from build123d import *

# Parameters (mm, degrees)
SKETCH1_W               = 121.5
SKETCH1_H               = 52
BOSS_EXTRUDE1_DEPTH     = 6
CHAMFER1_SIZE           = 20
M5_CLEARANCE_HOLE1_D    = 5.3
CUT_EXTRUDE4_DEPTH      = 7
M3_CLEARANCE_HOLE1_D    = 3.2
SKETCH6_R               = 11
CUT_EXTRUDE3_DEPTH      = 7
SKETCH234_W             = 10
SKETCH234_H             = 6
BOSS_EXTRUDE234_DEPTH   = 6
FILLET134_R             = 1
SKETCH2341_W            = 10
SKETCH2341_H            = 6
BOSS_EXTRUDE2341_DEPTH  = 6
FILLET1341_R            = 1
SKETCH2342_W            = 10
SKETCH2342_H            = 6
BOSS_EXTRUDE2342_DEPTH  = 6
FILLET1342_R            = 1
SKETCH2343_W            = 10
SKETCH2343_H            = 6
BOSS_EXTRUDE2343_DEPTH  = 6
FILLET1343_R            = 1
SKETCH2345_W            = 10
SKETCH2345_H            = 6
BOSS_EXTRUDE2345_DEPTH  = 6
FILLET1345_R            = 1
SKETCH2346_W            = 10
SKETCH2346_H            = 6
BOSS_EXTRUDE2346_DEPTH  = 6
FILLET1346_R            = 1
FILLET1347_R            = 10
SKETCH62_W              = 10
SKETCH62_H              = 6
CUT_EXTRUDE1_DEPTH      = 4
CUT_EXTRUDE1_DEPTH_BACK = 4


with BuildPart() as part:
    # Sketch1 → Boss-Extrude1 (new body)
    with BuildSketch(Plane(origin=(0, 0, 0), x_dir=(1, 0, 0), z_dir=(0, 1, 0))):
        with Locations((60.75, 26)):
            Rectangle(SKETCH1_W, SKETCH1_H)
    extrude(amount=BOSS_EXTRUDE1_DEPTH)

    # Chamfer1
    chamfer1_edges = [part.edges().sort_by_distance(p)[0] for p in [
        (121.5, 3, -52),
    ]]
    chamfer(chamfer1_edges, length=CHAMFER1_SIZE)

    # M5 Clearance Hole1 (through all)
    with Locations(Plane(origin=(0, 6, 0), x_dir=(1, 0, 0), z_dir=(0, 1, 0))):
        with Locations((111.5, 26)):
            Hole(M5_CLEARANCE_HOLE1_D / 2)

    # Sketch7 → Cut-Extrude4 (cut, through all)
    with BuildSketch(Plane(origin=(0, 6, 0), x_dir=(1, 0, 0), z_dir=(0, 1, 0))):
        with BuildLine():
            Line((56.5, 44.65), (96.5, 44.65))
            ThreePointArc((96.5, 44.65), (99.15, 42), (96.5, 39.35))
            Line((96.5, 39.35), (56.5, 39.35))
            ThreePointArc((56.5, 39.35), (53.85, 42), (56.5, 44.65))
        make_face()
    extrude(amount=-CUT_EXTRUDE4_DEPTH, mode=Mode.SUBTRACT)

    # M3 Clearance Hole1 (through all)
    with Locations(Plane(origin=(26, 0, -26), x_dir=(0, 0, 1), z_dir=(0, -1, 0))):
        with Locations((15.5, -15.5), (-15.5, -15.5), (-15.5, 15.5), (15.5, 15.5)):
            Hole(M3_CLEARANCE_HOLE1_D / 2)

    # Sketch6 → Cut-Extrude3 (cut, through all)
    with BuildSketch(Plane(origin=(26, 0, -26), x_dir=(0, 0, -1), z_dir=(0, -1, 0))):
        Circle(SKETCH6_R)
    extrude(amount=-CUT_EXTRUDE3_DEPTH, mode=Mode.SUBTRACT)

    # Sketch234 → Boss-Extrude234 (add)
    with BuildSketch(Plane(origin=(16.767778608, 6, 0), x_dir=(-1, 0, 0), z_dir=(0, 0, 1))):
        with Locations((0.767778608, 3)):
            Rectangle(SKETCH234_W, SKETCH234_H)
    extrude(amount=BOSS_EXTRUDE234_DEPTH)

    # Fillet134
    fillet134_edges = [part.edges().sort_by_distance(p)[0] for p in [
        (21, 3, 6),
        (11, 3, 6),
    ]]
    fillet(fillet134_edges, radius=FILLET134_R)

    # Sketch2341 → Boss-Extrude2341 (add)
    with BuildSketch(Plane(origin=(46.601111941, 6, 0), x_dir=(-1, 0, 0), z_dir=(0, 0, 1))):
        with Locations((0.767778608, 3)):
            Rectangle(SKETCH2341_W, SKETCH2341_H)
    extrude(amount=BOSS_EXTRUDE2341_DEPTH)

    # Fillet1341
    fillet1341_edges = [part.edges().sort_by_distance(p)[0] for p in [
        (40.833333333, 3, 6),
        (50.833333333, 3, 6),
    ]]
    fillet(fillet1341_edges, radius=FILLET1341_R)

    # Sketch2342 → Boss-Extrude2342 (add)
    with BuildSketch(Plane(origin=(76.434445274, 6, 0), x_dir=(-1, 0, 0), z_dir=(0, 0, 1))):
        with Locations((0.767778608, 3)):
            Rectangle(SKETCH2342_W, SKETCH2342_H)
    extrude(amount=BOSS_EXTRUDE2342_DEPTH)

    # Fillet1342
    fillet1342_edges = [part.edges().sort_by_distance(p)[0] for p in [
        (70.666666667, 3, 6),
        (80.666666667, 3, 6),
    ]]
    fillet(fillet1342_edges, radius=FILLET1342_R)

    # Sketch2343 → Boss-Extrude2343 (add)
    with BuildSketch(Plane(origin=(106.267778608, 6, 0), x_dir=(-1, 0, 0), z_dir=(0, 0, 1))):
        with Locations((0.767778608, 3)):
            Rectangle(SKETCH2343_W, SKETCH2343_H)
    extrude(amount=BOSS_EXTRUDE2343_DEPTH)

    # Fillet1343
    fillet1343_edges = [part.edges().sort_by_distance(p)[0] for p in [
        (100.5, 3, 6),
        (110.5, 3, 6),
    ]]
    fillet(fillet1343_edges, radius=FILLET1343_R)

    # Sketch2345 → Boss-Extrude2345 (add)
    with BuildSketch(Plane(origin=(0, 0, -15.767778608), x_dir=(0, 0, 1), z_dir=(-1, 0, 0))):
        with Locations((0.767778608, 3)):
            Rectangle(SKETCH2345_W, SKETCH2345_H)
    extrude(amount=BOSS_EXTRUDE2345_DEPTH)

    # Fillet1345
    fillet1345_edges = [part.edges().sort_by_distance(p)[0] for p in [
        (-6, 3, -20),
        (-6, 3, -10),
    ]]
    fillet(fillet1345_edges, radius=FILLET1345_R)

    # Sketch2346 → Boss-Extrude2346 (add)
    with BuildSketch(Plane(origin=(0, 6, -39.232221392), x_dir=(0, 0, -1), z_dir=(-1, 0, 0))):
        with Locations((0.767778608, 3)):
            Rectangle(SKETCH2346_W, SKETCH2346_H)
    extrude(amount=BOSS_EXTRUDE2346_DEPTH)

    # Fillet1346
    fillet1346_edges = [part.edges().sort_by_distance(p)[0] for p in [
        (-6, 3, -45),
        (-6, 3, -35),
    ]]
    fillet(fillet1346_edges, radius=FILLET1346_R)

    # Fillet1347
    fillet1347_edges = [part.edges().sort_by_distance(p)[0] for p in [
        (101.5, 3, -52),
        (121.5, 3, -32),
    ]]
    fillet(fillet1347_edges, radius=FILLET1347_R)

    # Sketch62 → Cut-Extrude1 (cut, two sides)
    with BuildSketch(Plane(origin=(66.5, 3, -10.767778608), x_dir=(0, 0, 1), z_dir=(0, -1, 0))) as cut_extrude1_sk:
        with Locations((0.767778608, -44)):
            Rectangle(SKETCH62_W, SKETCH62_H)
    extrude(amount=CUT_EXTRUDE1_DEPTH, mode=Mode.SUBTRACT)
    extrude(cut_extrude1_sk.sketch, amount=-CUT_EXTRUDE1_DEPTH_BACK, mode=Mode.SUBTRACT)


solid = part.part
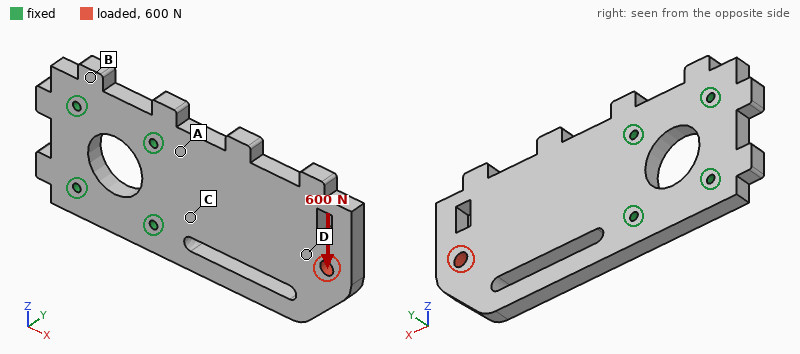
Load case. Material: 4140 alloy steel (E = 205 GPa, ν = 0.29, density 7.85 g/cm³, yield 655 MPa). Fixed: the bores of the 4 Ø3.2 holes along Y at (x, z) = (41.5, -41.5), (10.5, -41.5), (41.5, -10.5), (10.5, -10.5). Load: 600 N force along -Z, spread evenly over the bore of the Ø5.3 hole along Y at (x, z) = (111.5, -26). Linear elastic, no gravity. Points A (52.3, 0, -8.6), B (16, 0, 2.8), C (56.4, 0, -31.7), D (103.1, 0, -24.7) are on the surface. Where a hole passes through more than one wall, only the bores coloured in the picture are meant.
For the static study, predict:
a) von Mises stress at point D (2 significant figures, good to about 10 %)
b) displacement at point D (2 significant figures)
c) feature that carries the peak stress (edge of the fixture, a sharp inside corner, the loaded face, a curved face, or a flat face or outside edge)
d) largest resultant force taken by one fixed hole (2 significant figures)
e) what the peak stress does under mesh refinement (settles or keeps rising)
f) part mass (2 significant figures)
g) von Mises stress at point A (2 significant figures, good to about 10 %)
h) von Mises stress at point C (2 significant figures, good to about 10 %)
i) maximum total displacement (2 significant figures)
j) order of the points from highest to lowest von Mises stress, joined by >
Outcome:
4.4 MPa
8.6 µm
edge of the fixture
1.1 kN
keeps rising
270 g
11 MPa
8.0 MPa
12 µm
A > C > D > B
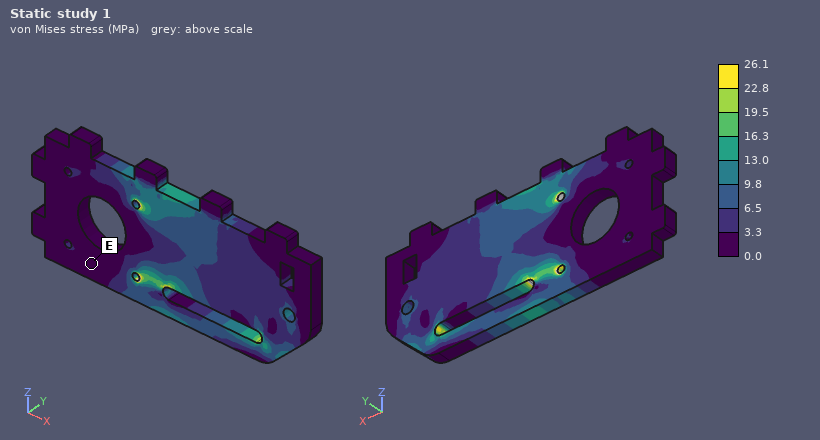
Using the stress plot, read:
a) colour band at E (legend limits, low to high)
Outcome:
0.0 to 3.3 MPa
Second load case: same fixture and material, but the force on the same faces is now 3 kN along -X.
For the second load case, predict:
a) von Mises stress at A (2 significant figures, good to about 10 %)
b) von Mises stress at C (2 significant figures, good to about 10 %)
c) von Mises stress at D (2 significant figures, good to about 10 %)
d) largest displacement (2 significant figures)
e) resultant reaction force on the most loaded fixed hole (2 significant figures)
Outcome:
11 MPa
11 MPa
25 MPa
6.7 µm
1.4 kN
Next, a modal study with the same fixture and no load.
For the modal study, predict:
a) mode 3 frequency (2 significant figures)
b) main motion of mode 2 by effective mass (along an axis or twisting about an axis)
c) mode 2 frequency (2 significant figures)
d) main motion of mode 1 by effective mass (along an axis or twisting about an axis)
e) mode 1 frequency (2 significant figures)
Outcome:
4600 Hz
twisting about X
2600 Hz
along Y
800 Hz
